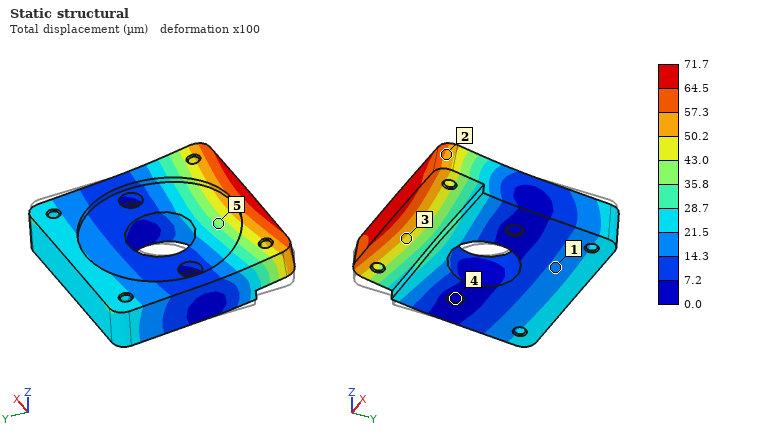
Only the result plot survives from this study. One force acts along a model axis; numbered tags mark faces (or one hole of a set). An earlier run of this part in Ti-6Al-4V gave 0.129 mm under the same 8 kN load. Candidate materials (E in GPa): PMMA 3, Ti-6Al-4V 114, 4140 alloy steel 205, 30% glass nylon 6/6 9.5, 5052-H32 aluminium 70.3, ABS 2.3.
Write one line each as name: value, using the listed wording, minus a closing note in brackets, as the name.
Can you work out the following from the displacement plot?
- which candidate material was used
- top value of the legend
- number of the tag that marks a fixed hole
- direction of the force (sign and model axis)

which candidate material was used: 4140 alloy steel
top value of the legend: 71.7 µm
number of the tag that marks a fixed hole: 4
direction of the force: +Z
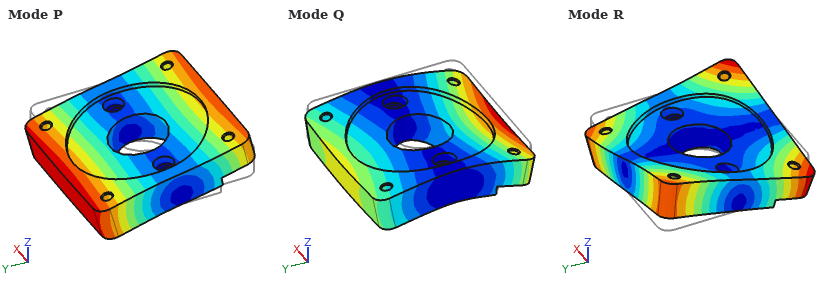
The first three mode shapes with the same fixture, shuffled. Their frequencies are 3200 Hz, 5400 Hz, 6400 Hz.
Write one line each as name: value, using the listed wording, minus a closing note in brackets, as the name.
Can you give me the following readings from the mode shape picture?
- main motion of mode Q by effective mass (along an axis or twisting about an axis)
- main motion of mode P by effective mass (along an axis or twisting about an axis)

main motion of mode Q by effective mass: along Z
main motion of mode P by effective mass: twisting about X
